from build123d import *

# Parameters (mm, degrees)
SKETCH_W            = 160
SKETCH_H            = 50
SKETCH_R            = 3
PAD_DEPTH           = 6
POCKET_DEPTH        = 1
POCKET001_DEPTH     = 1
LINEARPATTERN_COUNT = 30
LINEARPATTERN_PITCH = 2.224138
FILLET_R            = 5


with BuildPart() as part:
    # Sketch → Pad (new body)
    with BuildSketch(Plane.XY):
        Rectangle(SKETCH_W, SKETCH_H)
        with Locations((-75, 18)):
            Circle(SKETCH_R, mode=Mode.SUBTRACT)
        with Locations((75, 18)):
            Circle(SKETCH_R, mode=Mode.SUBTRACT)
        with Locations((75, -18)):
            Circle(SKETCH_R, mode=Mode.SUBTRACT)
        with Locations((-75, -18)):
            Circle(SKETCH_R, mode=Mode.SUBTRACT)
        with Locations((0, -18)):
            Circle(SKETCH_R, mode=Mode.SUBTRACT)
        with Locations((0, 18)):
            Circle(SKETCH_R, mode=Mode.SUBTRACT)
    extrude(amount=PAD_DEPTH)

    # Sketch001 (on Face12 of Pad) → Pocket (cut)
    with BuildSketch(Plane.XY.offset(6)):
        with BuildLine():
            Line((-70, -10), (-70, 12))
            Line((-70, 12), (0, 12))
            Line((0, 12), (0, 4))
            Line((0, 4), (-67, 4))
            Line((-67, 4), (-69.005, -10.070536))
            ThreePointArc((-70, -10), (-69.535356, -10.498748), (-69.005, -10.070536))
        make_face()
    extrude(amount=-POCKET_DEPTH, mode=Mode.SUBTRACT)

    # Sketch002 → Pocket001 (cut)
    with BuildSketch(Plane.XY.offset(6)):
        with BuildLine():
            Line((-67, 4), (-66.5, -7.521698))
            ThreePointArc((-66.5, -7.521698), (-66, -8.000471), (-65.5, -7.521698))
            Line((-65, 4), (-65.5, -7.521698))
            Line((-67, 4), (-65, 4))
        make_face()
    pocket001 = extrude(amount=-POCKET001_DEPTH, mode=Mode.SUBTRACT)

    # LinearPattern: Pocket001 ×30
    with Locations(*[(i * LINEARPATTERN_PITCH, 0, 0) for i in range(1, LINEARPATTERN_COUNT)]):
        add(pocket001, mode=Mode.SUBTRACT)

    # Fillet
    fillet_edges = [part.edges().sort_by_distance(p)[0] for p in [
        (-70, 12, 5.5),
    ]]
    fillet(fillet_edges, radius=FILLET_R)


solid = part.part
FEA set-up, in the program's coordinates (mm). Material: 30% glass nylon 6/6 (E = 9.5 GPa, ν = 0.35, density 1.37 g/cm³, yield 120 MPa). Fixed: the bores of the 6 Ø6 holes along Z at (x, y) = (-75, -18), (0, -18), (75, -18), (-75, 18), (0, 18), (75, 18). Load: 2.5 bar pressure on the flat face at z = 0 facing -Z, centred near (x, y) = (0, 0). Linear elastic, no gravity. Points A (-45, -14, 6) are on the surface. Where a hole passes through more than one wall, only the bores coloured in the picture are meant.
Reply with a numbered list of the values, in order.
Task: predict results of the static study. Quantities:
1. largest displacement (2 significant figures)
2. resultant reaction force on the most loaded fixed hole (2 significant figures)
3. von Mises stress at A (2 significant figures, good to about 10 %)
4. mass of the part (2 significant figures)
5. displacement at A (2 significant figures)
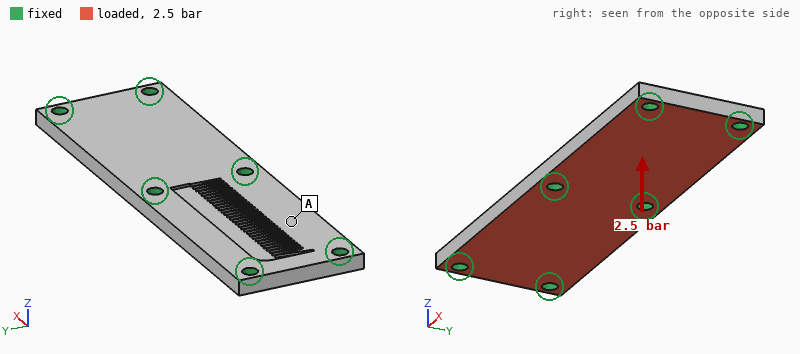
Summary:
1. 0.14 mm
2. 480 N
3. 9.1 MPa
4. 63 g
5. 0.12 mm
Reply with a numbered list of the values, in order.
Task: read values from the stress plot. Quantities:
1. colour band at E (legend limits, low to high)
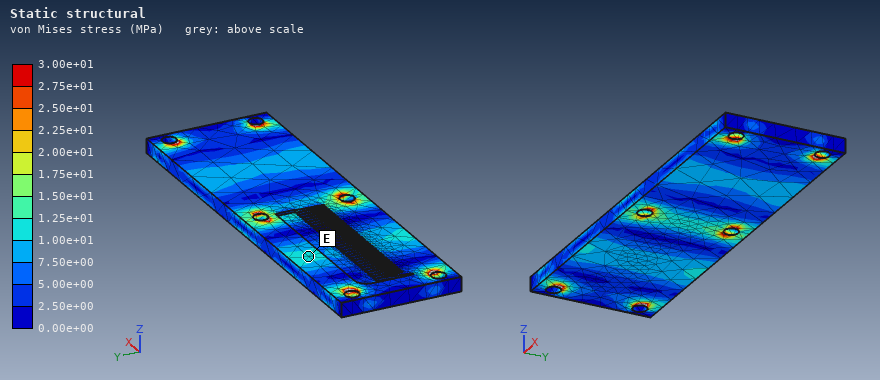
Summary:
1. 1.00e+01 to 1.25e+01 MPa
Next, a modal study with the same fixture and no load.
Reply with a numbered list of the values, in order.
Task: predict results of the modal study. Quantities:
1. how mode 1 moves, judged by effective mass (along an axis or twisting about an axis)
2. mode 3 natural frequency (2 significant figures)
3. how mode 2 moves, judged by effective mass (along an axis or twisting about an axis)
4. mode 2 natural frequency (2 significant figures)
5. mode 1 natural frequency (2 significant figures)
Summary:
1. twisting about Y
2. 3900 Hz
3. along Z
4. 2800 Hz
5. 2700 Hz
